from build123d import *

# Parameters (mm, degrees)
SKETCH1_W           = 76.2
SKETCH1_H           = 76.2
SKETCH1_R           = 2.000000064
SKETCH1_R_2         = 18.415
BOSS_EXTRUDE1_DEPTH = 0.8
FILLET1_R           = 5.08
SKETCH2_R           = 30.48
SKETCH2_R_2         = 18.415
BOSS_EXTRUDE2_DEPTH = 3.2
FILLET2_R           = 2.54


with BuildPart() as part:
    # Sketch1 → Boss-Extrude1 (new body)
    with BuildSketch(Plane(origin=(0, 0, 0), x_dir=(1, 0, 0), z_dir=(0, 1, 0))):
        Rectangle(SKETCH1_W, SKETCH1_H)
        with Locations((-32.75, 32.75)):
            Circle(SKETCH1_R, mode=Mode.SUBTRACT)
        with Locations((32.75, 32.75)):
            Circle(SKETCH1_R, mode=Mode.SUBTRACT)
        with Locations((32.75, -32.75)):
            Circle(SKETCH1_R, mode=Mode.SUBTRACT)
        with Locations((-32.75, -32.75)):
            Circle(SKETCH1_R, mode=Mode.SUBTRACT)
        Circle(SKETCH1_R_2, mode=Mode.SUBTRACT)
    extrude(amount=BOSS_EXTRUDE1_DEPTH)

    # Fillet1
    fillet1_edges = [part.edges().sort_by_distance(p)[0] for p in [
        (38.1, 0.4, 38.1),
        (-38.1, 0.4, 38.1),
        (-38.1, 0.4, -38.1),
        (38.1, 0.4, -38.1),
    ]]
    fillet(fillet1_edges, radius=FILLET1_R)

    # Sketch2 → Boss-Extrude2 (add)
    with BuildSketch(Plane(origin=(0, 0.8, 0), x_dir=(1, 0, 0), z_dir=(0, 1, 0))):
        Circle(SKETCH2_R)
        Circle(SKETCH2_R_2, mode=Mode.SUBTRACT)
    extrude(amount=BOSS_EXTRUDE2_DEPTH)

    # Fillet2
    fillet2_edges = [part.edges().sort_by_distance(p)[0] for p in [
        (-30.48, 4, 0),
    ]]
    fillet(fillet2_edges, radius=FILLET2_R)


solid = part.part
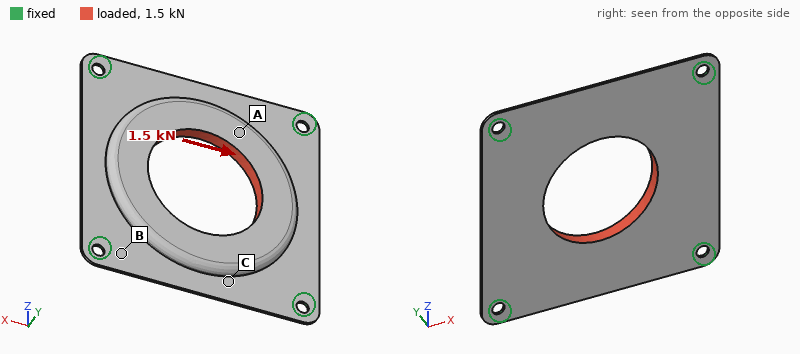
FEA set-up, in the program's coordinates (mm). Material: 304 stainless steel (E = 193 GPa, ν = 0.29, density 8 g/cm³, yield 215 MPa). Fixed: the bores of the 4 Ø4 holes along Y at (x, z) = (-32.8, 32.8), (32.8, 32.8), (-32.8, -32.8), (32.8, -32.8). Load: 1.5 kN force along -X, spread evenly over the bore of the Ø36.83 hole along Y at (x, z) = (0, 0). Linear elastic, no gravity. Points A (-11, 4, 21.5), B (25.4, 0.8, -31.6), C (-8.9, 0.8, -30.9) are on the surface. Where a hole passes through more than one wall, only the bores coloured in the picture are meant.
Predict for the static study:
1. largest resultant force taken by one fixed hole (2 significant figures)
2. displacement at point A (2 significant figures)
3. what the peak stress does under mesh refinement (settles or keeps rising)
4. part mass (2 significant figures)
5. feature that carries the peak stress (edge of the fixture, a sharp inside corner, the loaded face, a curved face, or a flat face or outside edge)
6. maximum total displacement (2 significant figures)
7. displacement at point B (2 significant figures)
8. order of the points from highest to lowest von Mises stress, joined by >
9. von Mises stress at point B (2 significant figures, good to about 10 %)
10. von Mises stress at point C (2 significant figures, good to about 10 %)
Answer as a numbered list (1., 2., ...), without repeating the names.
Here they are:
1. 400 N
2. 16 µm
3. keeps rising
4. 75 g
5. edge of the fixture
6. 49 µm
7. 8.7 µm
8. B > C > A
9. 46 MPa
10. 25 MPa
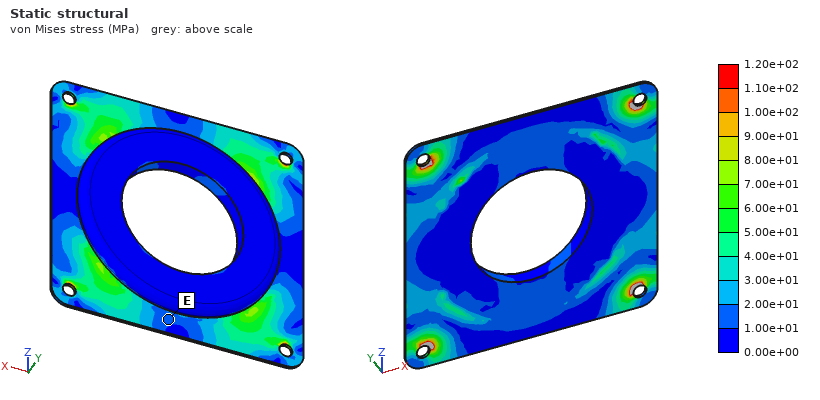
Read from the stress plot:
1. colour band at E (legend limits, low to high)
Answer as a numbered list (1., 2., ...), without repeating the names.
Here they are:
1. 1.00e+01 to 2.00e+01 MPa
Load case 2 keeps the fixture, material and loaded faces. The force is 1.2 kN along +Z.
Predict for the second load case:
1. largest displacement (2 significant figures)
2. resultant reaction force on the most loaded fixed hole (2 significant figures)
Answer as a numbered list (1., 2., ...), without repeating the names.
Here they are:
1. 39 µm
2. 320 N
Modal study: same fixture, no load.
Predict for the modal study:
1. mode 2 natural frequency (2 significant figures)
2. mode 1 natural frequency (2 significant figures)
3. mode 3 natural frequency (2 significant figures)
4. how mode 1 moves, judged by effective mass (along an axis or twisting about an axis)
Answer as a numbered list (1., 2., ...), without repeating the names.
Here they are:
1. 1300 Hz
2. 880 Hz
3. 1300 Hz
4. along Y
